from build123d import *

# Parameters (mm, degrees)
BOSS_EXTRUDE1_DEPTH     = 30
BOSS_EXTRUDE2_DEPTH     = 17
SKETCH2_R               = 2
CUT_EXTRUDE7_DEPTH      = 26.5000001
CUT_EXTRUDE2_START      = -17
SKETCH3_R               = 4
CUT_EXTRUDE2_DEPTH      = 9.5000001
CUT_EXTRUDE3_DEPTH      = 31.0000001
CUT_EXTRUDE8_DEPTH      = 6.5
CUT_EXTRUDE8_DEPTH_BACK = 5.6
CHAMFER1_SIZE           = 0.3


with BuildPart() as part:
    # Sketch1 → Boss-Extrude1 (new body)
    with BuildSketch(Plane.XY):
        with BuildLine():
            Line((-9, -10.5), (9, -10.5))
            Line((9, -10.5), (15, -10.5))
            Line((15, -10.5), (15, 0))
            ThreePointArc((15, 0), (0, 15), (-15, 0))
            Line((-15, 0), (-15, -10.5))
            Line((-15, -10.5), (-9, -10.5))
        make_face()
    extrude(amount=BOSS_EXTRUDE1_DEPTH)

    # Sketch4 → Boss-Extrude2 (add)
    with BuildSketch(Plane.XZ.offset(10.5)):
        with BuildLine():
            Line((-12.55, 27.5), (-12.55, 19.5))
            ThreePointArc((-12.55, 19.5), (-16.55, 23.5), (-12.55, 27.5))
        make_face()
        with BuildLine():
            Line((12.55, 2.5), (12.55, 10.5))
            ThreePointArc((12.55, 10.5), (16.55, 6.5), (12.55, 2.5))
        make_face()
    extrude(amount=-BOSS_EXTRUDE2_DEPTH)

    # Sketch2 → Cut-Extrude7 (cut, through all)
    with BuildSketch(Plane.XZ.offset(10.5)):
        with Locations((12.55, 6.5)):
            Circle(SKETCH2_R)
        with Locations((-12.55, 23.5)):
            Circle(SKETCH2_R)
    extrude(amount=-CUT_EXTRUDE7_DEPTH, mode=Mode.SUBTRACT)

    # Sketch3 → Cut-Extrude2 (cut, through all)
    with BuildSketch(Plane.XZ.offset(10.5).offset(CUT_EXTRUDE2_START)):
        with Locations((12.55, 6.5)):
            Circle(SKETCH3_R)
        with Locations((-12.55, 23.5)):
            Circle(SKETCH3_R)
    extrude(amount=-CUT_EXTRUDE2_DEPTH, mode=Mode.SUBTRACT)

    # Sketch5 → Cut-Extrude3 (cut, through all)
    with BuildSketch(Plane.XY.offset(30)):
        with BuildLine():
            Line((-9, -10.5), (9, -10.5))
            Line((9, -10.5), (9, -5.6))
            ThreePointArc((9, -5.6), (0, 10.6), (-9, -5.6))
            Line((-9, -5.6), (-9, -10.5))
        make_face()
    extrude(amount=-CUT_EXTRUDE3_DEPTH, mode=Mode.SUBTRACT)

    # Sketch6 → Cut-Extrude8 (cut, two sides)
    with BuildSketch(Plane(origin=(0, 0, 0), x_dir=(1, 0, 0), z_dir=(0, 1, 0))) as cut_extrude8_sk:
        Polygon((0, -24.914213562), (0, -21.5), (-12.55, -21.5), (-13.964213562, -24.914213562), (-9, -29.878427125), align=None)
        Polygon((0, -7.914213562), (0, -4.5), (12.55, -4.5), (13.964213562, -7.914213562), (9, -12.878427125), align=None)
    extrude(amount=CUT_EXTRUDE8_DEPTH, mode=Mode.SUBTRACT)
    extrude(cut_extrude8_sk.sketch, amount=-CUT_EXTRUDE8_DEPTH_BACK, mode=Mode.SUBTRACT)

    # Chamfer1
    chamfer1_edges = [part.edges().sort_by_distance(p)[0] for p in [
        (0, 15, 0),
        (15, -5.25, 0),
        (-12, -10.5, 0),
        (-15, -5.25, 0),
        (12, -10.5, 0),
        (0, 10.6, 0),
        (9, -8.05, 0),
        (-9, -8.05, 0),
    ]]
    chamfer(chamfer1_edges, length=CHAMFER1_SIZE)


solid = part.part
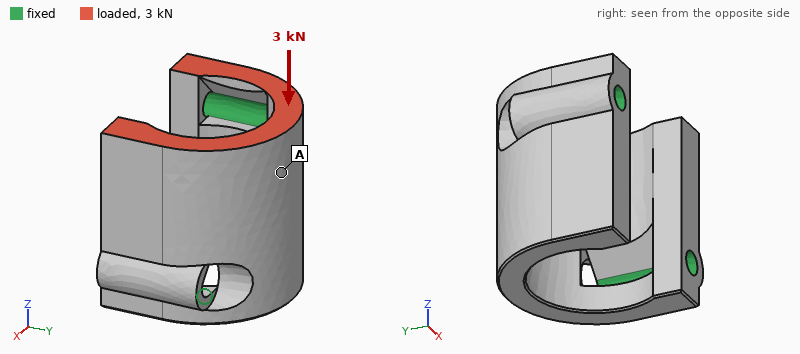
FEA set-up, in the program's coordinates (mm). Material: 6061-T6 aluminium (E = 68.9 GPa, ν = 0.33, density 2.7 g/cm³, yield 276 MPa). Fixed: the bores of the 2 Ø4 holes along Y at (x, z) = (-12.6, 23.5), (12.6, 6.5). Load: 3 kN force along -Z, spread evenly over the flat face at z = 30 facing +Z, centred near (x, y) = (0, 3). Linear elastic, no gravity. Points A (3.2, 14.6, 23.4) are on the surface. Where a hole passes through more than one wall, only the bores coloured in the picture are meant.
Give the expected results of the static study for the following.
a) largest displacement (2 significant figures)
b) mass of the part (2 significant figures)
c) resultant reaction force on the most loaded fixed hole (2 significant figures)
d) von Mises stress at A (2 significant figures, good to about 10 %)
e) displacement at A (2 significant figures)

31 µm
22 g
1.5 kN
13 MPa
26 µm
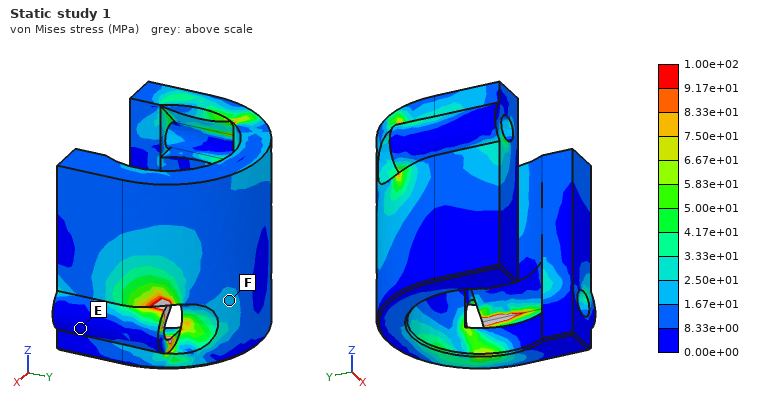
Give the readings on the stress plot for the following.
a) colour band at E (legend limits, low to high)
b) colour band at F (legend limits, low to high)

0.00e+00 to 8.33e+00 MPa
1.67e+01 to 2.50e+01 MPa
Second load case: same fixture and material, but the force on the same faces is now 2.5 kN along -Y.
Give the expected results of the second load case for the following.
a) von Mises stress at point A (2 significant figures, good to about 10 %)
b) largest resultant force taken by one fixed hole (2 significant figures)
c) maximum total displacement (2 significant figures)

29 MPa
1.4 kN
61 µm
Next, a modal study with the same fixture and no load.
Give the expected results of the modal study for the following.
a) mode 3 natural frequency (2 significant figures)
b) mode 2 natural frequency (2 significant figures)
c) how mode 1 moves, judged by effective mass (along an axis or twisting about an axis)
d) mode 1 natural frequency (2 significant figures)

14 kHz
12 kHz
along X
9200 Hz
